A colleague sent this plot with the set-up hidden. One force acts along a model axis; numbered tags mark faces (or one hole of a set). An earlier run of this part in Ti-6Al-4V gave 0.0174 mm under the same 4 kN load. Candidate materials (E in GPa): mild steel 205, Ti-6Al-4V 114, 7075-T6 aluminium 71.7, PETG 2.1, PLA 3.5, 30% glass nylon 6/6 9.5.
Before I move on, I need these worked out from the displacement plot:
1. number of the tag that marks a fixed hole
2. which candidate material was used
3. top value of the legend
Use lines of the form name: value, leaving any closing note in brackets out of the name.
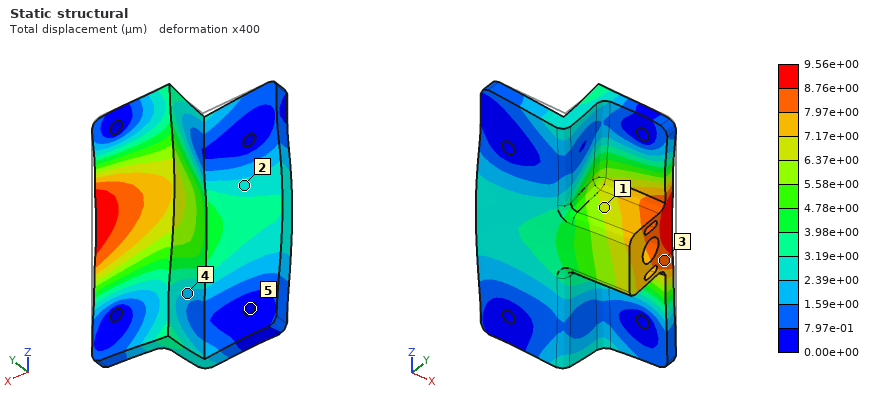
number of the tag that marks a fixed hole: 5
which candidate material was used: mild steel
top value of the legend: 9.56e+00 µm
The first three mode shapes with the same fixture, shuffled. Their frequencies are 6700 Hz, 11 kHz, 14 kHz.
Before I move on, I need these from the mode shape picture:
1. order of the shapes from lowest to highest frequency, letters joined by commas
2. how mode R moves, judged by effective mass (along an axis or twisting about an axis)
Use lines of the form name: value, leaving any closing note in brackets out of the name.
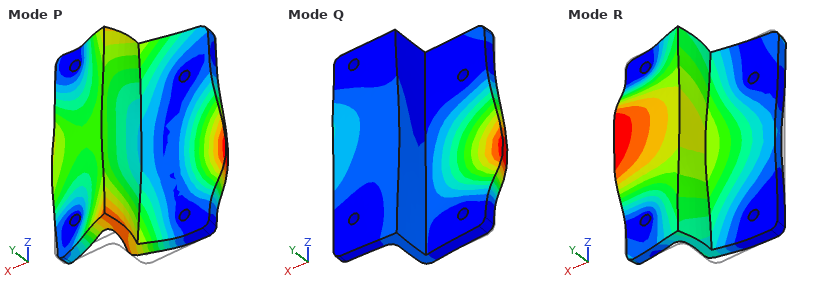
order of the shapes from lowest to highest frequency, letters joined by commas: R, Q, P
how mode R moves, judged by effective mass: along Y
